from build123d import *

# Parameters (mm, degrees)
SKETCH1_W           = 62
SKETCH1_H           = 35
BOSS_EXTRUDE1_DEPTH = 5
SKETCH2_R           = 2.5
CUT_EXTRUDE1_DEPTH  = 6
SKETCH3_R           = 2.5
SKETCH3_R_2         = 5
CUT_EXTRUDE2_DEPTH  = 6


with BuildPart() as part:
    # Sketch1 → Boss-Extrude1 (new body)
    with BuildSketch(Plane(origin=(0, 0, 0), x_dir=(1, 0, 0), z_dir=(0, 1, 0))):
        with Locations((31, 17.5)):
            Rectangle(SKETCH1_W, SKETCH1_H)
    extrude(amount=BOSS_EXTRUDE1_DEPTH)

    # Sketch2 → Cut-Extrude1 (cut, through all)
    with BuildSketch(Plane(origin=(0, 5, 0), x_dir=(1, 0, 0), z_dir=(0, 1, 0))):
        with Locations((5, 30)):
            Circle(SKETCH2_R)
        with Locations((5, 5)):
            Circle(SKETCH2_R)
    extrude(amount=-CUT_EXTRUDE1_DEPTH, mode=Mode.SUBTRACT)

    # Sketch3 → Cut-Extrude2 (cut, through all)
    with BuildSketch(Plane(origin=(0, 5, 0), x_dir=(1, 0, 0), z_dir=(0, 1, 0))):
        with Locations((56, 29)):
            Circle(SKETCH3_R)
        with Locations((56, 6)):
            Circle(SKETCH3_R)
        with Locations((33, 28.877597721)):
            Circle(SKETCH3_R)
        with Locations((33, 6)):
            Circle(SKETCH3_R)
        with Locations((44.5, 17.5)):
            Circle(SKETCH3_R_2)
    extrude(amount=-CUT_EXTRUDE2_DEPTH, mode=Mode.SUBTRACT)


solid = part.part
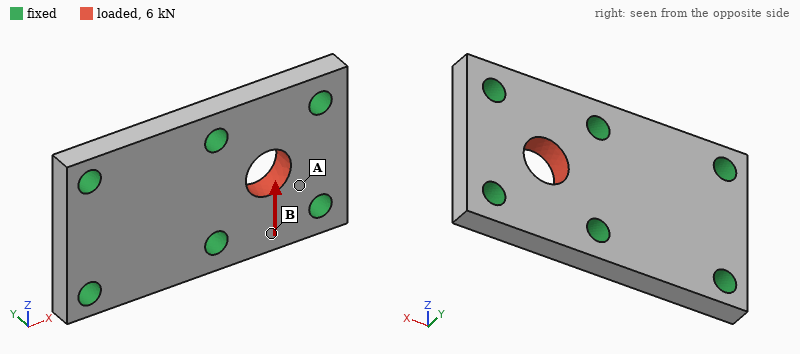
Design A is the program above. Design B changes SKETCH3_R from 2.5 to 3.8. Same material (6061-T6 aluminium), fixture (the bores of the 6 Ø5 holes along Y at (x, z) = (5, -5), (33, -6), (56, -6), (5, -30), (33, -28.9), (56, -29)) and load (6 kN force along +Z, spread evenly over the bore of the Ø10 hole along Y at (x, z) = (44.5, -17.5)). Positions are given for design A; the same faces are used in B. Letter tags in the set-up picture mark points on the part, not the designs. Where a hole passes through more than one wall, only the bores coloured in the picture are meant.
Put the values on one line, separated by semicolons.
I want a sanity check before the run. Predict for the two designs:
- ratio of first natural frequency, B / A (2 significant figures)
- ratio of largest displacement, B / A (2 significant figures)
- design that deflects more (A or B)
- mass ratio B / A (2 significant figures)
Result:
1.1; 0.83; A; 0.95
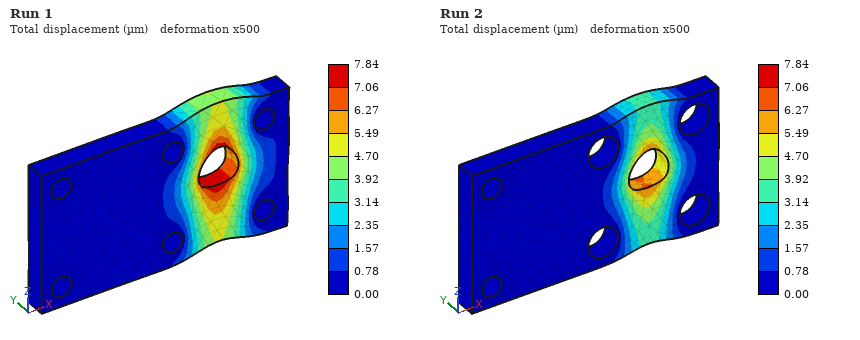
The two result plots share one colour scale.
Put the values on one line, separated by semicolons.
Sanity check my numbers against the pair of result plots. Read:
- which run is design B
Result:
Run 2
